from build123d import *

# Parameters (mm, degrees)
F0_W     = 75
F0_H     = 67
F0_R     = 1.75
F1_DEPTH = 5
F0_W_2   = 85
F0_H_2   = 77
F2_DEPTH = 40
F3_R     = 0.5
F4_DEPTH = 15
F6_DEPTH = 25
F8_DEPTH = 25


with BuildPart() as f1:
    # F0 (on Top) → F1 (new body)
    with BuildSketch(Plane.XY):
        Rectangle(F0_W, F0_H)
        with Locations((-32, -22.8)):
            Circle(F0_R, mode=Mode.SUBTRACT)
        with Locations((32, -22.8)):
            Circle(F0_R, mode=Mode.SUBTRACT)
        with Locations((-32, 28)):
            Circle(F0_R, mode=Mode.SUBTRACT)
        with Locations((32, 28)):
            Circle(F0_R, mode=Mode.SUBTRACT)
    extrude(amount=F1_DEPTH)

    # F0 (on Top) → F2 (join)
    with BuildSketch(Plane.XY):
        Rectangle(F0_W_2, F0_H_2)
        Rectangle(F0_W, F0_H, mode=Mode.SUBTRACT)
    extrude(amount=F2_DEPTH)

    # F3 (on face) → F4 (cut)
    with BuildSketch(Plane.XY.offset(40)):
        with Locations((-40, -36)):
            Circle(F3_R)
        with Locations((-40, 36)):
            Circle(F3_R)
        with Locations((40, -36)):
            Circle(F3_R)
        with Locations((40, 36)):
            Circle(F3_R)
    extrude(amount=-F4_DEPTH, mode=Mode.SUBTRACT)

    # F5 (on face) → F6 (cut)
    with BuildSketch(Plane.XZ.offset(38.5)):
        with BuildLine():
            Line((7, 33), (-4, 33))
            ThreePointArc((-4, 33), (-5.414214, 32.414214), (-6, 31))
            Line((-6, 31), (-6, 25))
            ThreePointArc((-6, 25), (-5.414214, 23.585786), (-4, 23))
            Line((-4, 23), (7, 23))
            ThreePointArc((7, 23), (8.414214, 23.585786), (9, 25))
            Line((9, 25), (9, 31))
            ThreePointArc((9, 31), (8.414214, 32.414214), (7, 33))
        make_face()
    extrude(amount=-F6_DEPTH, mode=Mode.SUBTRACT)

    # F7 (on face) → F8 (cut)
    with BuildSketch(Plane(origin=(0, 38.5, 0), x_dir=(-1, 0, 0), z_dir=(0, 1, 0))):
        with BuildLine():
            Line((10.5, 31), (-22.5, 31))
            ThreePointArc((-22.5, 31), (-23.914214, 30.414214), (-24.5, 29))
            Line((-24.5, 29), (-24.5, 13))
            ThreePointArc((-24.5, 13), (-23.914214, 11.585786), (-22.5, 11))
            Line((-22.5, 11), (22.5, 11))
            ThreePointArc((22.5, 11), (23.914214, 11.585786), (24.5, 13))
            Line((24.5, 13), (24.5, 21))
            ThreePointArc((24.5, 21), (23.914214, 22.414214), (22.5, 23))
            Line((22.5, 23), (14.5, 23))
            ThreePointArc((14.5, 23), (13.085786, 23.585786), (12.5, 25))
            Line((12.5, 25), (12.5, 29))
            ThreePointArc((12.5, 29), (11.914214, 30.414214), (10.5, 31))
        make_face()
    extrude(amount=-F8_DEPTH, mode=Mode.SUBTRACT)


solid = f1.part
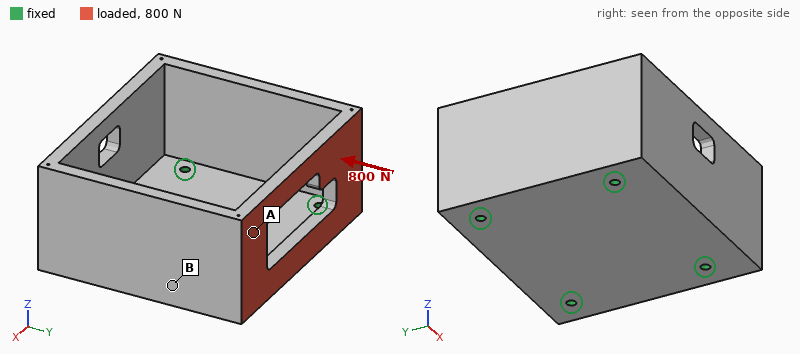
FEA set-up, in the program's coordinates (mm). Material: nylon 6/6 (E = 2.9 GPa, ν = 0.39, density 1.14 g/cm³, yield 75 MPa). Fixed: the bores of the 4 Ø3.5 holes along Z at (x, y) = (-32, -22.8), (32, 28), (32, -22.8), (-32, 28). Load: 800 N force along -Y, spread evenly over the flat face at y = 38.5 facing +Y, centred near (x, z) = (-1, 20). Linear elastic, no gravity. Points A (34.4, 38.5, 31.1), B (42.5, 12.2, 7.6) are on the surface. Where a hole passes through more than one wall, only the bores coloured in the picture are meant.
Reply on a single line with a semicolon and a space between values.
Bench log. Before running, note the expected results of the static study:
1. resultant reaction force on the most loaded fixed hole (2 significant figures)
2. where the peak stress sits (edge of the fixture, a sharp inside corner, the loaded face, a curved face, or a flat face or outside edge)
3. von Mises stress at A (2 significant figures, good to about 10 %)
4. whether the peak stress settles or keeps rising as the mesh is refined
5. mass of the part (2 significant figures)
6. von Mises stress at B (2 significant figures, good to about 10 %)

270 N; a sharp inside corner; 12 MPa; keeps rising; 92 g; 2.9 MPa
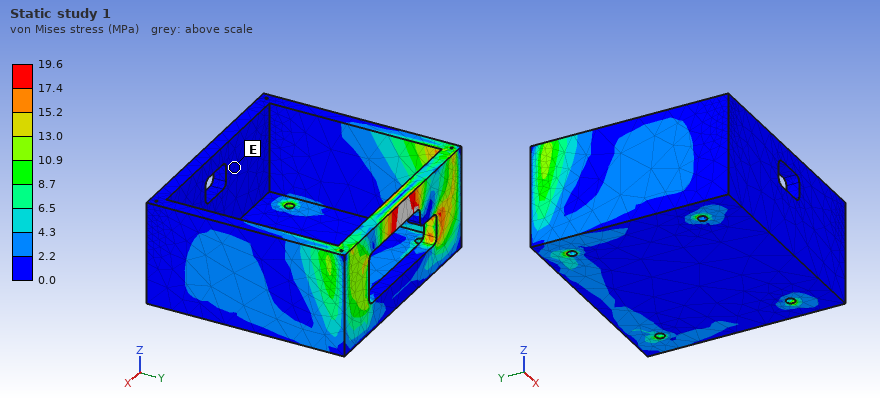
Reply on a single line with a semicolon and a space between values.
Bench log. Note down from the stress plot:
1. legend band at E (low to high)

0.0 to 2.2 MPa
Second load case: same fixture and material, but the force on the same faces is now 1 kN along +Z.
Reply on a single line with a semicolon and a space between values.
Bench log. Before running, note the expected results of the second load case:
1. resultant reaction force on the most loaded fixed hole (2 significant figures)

600 N
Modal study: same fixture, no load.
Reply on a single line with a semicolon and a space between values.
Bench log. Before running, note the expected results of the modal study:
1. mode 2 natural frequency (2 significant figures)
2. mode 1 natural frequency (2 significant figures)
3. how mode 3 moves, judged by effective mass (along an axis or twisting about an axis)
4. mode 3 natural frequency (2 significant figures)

1300 Hz; 1200 Hz; along Y; 1400 Hz
